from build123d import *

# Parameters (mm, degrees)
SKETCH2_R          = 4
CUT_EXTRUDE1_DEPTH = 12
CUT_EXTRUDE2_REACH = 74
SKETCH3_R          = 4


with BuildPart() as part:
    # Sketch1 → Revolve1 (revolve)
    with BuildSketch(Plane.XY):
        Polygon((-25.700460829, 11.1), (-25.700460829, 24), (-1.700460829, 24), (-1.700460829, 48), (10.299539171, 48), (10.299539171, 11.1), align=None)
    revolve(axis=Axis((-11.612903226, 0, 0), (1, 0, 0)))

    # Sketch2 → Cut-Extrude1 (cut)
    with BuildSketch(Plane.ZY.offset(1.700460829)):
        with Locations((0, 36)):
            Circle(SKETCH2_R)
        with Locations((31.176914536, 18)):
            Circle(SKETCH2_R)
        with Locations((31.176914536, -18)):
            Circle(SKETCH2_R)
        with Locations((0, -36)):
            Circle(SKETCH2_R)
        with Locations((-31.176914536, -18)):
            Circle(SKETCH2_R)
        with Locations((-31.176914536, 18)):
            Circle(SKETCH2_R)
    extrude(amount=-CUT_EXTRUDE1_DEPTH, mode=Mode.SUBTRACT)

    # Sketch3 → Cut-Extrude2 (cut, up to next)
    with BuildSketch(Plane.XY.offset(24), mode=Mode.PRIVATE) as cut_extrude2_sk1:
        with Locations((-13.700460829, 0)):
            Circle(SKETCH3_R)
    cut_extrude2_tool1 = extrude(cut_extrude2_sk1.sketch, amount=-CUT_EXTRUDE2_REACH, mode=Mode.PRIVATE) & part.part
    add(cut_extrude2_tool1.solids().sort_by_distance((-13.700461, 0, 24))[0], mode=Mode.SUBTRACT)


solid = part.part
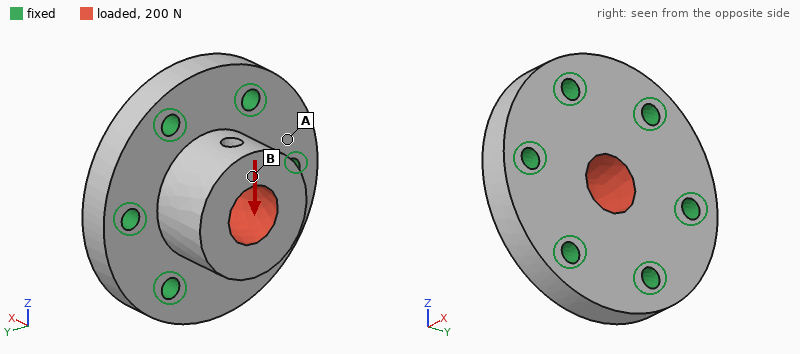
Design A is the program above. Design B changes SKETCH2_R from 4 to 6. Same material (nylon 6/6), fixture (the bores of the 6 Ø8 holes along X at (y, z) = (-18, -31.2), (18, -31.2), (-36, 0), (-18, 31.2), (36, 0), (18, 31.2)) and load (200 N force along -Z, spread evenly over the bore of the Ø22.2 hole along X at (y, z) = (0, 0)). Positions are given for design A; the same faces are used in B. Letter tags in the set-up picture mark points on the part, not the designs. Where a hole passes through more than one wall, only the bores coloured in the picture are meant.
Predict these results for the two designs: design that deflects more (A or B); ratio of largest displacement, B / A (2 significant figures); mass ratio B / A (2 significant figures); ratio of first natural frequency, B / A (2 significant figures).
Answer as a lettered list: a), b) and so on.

a) A
b) 0.90
c) 0.96
d) 1.1
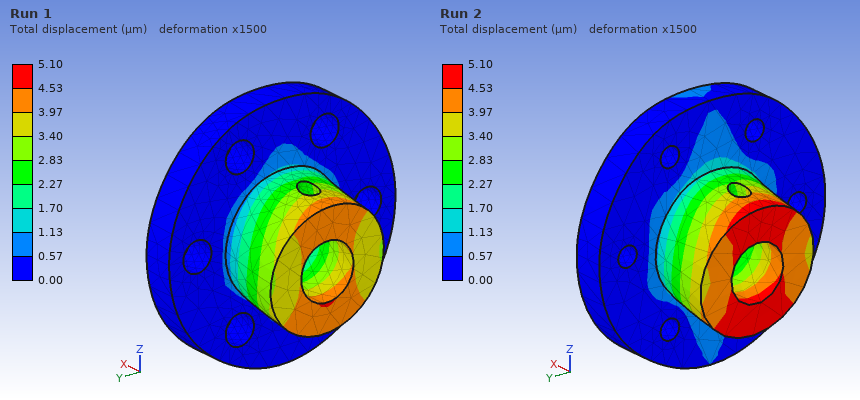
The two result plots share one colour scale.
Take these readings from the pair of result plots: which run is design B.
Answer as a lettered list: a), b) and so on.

a) Run 1
